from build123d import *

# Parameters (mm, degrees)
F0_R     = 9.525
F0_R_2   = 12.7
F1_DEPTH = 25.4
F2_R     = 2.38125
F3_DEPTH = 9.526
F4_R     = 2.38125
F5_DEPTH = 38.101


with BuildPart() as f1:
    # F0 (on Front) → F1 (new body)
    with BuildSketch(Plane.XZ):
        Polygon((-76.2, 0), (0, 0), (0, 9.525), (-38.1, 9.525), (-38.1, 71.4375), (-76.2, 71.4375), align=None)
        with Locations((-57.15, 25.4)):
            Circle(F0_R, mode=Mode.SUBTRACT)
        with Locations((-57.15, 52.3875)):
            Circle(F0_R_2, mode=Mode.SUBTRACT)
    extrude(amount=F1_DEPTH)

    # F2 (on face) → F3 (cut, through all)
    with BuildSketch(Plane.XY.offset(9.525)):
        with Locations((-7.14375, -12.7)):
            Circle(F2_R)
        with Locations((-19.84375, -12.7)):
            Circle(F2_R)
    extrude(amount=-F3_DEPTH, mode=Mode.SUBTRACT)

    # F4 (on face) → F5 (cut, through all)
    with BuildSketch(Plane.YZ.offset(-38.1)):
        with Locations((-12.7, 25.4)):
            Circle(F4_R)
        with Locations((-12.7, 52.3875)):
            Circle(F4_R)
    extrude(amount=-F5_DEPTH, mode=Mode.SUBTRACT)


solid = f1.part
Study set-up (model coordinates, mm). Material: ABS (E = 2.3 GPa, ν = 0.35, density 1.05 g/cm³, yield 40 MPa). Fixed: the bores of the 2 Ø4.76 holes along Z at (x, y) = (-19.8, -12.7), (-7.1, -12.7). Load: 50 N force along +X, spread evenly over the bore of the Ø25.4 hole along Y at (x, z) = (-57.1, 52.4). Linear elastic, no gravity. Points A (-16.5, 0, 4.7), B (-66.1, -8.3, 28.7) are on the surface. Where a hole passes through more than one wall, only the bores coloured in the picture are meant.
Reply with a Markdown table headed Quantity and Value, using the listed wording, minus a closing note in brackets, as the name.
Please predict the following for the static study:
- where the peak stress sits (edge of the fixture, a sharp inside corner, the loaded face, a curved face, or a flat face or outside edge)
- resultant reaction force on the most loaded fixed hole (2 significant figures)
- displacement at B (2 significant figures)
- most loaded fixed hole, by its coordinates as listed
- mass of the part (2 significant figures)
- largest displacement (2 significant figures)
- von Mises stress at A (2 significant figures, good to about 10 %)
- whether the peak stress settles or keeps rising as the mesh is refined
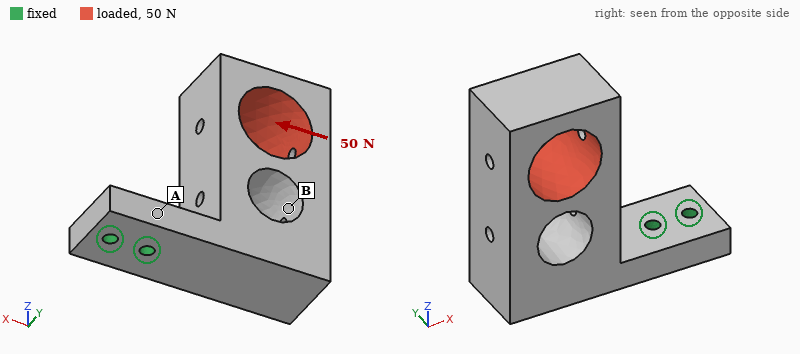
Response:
| Quantity | Value |
|---|---|
| where the peak stress sits | edge of the fixture |
| resultant reaction force on the most loaded fixed hole | 72 N |
| displacement at B | 0.58 mm |
| most loaded fixed hole, by its coordinates as listed | (-19.8, -12.7) |
| mass of the part | 60 g |
| largest displacement | 1.1 mm |
| von Mises stress at A | 1.6 MPa |
| whether the peak stress settles or keeps rising as the mesh is refined | keeps rising |
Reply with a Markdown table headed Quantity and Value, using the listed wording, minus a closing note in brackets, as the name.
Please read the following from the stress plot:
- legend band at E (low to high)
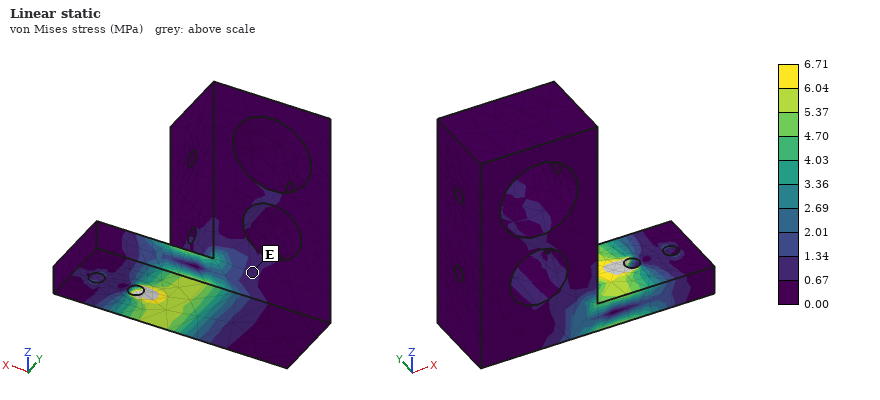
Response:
| Quantity | Value |
|---|---|
| legend band at E | 0.67 to 1.34 MPa |
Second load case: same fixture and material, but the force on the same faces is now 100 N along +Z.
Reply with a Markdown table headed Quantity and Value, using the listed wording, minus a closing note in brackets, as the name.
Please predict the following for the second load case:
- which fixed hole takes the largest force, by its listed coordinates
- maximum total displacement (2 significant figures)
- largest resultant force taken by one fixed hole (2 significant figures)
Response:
| Quantity | Value |
|---|---|
| which fixed hole takes the largest force, by its listed coordinates | (-19.8, -12.7) |
| maximum total displacement | 1.2 mm |
| largest resultant force taken by one fixed hole | 180 N |
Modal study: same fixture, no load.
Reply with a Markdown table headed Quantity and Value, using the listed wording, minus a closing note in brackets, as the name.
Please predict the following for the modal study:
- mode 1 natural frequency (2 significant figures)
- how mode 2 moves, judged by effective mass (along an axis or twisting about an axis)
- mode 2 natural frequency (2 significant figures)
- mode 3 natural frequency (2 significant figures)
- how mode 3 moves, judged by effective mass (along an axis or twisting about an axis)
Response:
| Quantity | Value |
|---|---|
| mode 1 natural frequency | 200 Hz |
| how mode 2 moves, judged by effective mass | along Y |
| mode 2 natural frequency | 280 Hz |
| mode 3 natural frequency | 800 Hz |
| how mode 3 moves, judged by effective mass | along Y |
